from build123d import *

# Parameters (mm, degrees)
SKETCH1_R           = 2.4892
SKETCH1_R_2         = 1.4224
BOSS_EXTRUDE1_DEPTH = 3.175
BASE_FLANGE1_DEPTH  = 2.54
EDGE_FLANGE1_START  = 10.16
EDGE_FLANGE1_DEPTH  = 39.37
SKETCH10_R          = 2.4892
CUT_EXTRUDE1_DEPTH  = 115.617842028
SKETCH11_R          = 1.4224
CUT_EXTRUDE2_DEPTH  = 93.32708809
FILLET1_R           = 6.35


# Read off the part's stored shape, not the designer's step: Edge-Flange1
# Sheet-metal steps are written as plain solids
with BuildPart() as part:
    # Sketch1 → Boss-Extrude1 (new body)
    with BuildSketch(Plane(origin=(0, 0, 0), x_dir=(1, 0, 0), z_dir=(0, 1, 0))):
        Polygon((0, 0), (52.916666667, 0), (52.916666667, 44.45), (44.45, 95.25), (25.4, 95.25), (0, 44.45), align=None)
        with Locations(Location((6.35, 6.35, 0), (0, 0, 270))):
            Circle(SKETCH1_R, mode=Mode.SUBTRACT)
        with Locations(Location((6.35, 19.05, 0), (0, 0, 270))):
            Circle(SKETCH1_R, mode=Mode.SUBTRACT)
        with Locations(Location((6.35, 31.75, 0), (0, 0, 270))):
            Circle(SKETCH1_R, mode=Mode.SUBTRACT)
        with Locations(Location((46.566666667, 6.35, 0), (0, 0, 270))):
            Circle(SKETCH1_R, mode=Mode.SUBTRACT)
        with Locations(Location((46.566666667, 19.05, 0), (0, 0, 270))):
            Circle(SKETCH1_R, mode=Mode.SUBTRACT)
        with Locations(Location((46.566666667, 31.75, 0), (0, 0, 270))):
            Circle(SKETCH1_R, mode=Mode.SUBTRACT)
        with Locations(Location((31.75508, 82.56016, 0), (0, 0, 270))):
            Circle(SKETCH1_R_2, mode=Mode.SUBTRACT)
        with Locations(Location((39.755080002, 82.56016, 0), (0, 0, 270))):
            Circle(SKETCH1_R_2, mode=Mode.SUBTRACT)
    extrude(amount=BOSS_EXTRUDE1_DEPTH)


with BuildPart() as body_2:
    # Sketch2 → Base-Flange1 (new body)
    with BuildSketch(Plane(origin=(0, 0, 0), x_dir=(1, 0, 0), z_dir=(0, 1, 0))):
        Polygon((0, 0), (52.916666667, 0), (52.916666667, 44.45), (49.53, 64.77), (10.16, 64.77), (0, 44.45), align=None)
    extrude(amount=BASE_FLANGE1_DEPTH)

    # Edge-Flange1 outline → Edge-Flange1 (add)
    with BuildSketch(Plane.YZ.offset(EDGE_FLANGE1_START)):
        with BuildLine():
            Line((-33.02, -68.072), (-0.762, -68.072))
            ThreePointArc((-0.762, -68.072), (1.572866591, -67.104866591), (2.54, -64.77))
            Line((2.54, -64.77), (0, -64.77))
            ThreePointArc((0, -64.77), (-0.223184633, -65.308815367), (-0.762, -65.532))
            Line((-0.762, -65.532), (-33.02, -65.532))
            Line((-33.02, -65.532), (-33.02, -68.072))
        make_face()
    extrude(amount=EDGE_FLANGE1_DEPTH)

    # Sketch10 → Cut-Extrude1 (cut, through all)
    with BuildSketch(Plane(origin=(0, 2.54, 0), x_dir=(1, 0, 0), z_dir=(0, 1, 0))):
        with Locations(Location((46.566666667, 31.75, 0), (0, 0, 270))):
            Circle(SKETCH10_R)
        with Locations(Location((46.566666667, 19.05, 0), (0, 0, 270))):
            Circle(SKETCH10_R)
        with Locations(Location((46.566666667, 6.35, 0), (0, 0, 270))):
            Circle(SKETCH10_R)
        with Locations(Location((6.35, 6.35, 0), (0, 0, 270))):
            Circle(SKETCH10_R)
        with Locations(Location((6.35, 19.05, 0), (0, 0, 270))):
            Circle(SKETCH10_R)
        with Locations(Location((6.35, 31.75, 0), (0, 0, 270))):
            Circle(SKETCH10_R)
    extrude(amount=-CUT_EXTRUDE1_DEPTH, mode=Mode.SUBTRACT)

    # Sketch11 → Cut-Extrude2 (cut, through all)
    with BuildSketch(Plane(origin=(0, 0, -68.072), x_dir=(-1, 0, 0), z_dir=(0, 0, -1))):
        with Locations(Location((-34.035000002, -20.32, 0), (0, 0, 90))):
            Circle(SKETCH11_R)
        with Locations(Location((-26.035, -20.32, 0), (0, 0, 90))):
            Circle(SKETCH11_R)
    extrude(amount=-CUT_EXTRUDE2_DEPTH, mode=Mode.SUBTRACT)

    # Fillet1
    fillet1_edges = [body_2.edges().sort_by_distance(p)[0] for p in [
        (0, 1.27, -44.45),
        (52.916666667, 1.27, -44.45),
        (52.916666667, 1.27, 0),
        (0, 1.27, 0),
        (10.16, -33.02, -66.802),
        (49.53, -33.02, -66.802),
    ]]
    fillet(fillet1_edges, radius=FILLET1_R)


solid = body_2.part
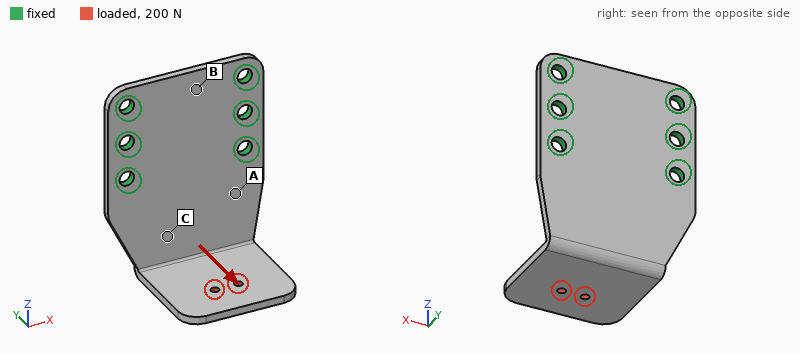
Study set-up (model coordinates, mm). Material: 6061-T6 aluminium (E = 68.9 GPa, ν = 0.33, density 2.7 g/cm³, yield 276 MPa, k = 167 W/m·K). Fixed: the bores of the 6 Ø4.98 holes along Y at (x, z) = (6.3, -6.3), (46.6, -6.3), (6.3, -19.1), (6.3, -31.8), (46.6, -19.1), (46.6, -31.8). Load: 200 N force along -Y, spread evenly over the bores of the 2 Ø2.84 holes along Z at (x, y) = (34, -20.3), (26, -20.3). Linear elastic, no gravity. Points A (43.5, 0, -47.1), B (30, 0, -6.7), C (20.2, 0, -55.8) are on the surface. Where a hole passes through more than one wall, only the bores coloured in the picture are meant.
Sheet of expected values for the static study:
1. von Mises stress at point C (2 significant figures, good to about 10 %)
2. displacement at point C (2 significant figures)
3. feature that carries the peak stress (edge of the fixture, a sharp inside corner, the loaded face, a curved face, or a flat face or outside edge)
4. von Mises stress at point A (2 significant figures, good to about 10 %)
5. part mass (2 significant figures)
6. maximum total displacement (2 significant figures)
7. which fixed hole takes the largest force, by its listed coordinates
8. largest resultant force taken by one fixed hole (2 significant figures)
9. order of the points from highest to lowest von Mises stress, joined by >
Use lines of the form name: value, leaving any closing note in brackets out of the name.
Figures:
von Mises stress at point C: 44 MPa
displacement at point C: 0.33 mm
feature that carries the peak stress: a flat face or outside edge
von Mises stress at point A: 70 MPa
part mass: 31 g
maximum total displacement: 1.1 mm
which fixed hole takes the largest force, by its listed coordinates: (46.6, -31.8)
largest resultant force taken by one fixed hole: 190 N
order of the points from highest to lowest von Mises stress, joined by >: A > C > B
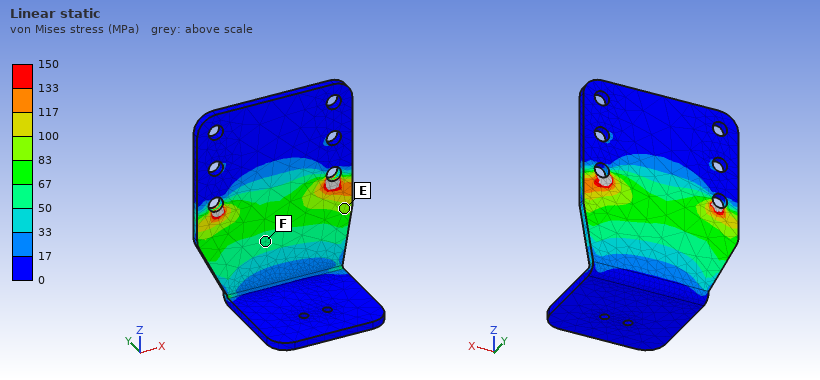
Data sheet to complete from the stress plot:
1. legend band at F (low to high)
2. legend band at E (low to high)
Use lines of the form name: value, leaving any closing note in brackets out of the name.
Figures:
legend band at F: 50 to 67 MPa
legend band at E: 83 to 100 MPa
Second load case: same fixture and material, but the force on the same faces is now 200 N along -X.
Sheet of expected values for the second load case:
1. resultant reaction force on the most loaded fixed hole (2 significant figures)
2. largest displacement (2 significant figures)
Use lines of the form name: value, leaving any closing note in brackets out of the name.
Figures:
resultant reaction force on the most loaded fixed hole: 210 N
largest displacement: 0.48 mm
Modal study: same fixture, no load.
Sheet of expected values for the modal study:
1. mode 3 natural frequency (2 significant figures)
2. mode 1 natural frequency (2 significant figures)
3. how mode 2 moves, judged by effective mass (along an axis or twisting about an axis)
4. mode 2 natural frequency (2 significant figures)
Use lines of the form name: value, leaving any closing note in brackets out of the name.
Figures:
mode 3 natural frequency: 1700 Hz
mode 1 natural frequency: 670 Hz
how mode 2 moves, judged by effective mass: along X
mode 2 natural frequency: 1300 Hz
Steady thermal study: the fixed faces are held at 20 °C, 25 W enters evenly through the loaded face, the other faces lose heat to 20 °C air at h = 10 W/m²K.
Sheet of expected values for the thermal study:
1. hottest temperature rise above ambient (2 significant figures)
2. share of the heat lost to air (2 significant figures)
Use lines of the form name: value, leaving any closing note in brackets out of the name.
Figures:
hottest temperature rise above ambient: 82 K
share of the heat lost to air: 10 %
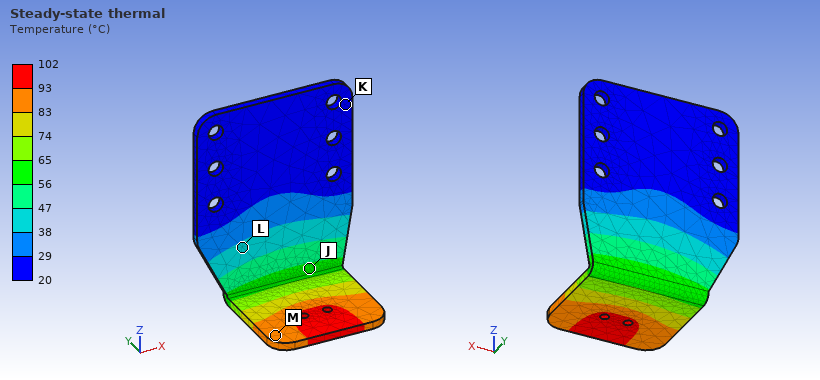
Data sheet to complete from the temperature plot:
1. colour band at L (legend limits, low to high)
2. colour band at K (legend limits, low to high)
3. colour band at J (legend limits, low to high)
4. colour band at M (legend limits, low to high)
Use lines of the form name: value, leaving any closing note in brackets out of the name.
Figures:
colour band at L: 38 to 47 °C
colour band at K: 20 to 29 °C
colour band at J: 56 to 65 °C
colour band at M: 83 to 93 °C
